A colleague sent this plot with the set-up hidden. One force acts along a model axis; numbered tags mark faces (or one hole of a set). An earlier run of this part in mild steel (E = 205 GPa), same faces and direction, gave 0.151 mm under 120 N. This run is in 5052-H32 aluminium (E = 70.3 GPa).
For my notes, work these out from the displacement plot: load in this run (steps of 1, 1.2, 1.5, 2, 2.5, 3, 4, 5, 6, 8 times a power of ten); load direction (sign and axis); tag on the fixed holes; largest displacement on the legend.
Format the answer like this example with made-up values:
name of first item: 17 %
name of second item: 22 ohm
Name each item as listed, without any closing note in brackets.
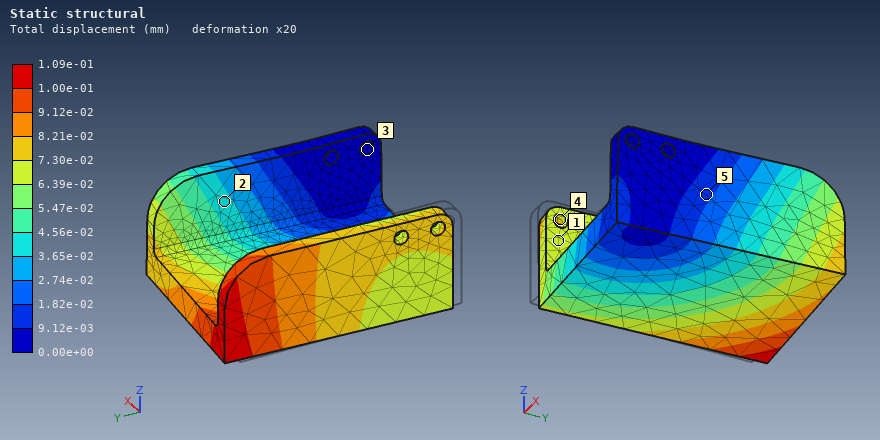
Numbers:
load in this run: 30 N
load direction: +Y
tag on the fixed holes: 3
largest displacement on the legend: 1.09e-01 mm
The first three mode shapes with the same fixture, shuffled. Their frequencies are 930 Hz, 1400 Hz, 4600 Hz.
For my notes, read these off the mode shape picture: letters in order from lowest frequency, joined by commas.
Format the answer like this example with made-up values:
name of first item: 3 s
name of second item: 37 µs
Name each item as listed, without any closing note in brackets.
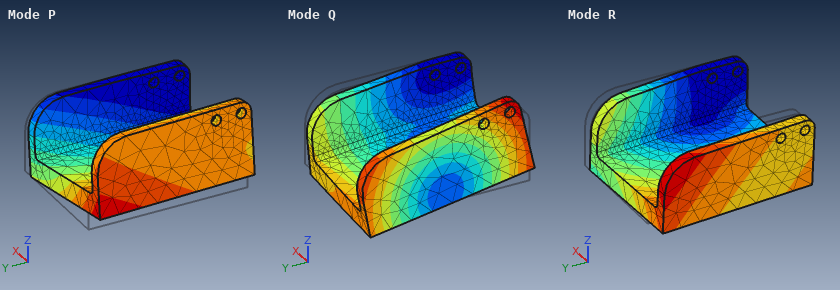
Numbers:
letters in order from lowest frequency, joined by commas: P, R, Q
